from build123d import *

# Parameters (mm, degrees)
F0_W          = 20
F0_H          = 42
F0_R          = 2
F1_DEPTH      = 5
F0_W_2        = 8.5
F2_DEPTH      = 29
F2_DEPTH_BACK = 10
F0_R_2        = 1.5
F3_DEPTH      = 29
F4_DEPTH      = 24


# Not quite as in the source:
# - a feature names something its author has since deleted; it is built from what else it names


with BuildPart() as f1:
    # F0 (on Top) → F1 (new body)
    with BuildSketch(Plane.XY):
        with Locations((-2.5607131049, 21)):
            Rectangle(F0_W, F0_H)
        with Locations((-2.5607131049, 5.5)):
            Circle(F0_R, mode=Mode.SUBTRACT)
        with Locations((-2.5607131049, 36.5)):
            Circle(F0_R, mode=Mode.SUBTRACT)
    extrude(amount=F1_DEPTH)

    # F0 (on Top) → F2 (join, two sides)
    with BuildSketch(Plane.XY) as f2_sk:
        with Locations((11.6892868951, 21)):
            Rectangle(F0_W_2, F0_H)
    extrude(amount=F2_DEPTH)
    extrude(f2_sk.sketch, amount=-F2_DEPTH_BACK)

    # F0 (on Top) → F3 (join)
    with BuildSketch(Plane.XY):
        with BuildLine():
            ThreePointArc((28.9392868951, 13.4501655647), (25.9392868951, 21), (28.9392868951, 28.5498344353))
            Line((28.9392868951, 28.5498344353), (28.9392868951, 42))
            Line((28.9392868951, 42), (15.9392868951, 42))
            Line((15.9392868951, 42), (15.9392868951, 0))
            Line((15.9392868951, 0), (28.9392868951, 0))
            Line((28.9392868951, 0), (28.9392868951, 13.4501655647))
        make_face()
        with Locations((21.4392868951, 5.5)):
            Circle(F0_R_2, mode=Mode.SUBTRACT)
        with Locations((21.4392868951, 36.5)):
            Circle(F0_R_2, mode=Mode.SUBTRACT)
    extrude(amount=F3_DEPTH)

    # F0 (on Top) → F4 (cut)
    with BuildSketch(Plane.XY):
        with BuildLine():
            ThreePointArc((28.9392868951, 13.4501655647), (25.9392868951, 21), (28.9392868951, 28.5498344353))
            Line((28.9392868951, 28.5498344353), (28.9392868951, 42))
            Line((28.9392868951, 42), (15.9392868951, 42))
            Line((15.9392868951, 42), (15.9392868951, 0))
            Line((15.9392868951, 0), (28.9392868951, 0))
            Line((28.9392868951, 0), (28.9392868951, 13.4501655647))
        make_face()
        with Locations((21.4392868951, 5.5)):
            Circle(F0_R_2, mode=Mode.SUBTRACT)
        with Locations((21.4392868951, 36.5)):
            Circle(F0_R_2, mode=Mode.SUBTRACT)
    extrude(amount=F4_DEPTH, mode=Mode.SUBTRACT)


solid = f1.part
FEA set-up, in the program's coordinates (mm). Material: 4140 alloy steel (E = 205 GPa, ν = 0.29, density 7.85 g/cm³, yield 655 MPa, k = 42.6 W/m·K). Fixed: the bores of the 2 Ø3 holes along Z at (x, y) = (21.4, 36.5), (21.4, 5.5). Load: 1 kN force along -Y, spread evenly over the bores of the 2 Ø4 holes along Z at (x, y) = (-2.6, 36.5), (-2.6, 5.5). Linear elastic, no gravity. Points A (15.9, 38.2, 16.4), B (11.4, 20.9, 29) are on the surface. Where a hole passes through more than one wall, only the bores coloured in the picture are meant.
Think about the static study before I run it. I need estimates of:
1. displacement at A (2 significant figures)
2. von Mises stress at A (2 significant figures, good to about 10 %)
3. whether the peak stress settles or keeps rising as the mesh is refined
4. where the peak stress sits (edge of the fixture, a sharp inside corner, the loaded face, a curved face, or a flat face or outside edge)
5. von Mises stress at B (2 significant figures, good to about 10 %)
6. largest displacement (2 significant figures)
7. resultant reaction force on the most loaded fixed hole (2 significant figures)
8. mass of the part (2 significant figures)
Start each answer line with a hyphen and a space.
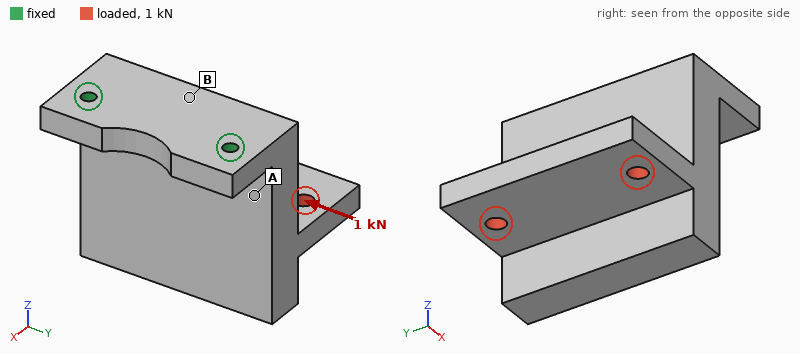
- 4.1 µm
- 15 MPa
- keeps rising
- edge of the fixture
- 7.0 MPa
- 14 µm
- 1.2 kN
- 160 g
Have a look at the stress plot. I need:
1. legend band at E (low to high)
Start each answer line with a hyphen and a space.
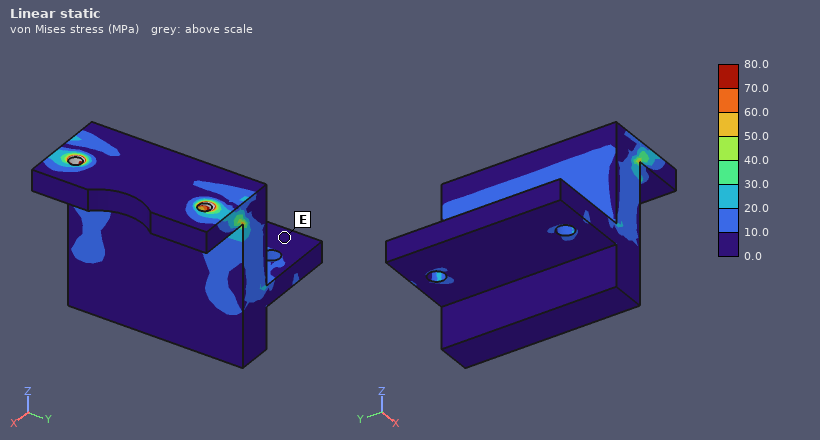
- 0.0 to 10.0 MPa
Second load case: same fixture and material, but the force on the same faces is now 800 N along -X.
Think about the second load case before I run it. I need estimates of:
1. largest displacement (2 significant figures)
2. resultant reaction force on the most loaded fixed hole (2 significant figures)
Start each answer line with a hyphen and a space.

- 0.10 mm
- 420 N
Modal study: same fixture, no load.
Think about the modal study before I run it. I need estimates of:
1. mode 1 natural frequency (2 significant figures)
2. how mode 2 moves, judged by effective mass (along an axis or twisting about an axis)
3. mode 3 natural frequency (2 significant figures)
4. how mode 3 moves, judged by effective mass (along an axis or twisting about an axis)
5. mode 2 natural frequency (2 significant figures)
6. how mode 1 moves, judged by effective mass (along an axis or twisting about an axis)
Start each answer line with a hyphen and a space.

- 1500 Hz
- along Y
- 6300 Hz
- along Y
- 5400 Hz
- along X
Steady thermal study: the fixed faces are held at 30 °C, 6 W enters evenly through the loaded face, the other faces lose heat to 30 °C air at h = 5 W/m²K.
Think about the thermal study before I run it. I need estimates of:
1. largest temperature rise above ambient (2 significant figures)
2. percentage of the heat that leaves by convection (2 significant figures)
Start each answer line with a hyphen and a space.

- 26 K
- 8.2 %
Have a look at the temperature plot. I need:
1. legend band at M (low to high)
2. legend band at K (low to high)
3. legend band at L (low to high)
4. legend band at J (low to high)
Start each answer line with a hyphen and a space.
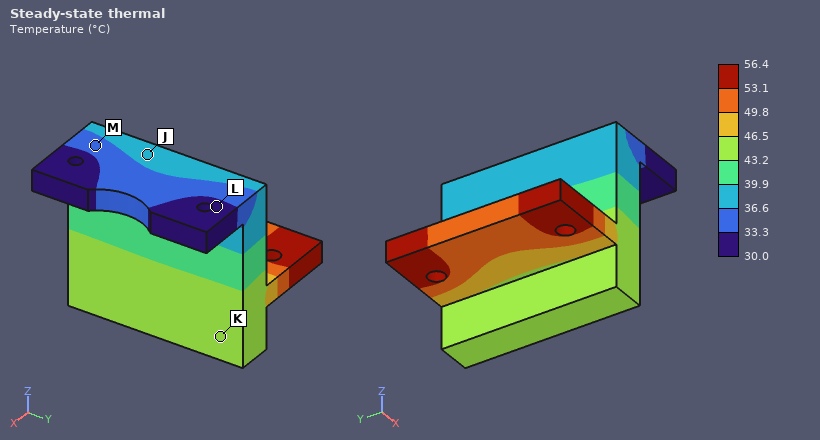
- 33.3 to 36.6 °C
- 43.2 to 46.5 °C
- 30.0 to 33.3 °C
- 36.6 to 39.9 °C
